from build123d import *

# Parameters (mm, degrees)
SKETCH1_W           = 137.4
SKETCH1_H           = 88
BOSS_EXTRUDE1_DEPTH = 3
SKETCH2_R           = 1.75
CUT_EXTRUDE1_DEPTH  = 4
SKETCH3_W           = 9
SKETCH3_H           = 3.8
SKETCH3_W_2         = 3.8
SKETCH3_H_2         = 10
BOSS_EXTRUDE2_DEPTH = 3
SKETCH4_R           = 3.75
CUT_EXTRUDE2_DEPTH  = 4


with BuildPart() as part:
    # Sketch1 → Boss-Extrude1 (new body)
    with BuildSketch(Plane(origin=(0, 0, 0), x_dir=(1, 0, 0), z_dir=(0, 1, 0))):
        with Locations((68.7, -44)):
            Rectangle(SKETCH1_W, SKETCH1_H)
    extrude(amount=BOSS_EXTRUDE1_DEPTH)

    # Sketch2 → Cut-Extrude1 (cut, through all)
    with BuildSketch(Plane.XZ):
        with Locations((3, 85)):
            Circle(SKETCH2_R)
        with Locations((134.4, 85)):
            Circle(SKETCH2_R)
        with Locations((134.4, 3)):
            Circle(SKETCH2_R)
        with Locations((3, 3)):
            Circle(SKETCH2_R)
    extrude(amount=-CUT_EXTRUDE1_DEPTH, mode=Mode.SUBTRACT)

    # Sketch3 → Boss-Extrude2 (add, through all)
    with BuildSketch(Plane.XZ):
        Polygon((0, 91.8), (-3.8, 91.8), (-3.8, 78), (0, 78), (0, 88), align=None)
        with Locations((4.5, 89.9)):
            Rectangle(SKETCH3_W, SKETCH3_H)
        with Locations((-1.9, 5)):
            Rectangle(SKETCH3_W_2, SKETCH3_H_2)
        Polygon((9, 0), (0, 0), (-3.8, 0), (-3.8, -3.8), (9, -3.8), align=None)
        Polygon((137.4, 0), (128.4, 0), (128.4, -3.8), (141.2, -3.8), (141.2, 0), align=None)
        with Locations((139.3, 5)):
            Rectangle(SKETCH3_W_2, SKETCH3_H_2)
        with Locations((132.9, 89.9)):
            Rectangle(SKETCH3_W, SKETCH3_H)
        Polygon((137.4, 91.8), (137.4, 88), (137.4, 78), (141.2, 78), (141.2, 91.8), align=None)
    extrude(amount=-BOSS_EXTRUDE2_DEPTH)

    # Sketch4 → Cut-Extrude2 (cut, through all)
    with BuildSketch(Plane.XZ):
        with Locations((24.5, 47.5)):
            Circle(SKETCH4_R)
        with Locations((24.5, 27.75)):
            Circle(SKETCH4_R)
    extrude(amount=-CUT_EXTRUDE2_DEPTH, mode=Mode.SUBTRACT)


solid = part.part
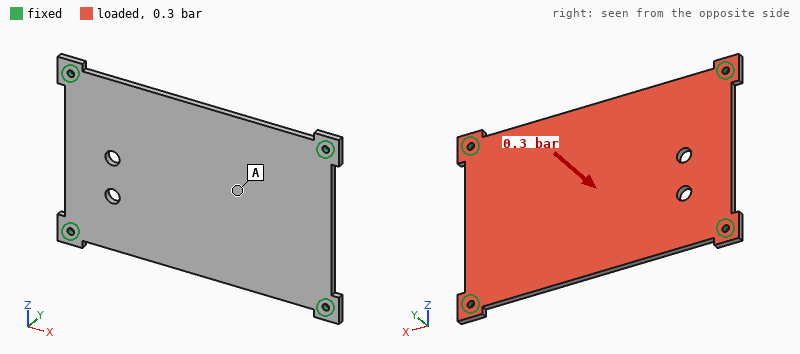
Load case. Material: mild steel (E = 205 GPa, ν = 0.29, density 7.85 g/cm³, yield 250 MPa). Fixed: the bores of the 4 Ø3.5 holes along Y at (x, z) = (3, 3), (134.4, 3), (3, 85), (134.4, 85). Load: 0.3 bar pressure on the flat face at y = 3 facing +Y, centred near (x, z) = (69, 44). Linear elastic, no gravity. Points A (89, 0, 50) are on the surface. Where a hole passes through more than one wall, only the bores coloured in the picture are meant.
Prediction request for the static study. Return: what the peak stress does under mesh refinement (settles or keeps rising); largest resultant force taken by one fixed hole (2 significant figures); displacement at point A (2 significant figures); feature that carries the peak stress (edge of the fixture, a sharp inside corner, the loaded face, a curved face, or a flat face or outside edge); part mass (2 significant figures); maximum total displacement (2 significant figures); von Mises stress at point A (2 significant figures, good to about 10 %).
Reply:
keeps rising
93 N
78 µm
edge of the fixture
290 g
89 µm
13 MPa
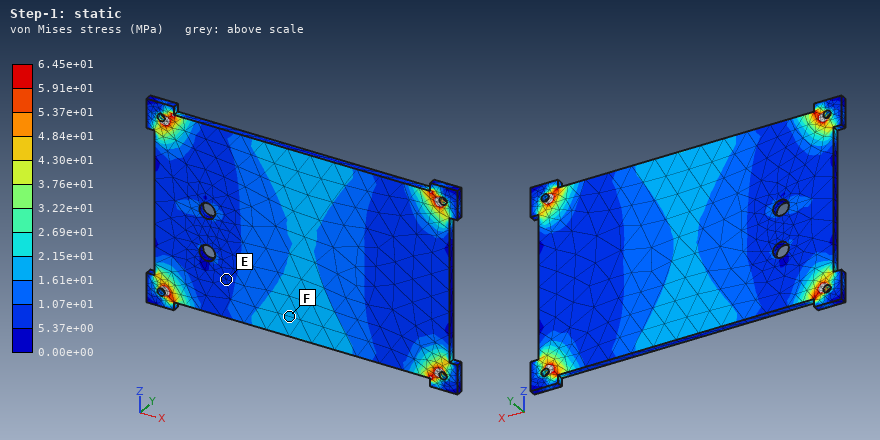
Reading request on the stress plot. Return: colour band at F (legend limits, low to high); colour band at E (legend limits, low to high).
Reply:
1.61e+01 to 2.15e+01 MPa
5.37e+00 to 1.07e+01 MPa
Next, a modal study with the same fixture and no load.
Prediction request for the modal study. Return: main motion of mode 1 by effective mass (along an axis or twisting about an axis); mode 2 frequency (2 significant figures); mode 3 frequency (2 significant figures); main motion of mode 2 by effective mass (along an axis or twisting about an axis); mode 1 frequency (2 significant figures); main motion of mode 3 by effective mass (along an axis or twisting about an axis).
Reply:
along Y
1200 Hz
1800 Hz
twisting about X
690 Hz
twisting about Z
